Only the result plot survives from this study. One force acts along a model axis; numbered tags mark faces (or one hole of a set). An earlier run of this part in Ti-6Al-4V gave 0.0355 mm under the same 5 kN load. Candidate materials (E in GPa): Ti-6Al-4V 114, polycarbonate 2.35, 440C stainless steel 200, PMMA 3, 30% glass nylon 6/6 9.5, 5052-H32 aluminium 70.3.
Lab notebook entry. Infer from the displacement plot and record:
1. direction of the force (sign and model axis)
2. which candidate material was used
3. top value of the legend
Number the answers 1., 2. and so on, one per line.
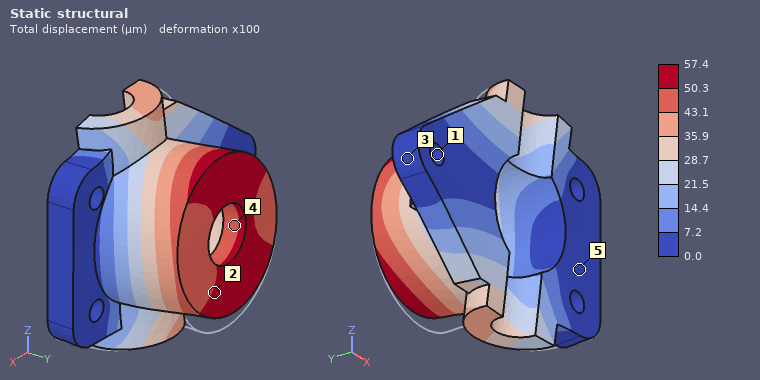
1. +Z
2. 5052-H32 aluminium
3. 57.4 µm
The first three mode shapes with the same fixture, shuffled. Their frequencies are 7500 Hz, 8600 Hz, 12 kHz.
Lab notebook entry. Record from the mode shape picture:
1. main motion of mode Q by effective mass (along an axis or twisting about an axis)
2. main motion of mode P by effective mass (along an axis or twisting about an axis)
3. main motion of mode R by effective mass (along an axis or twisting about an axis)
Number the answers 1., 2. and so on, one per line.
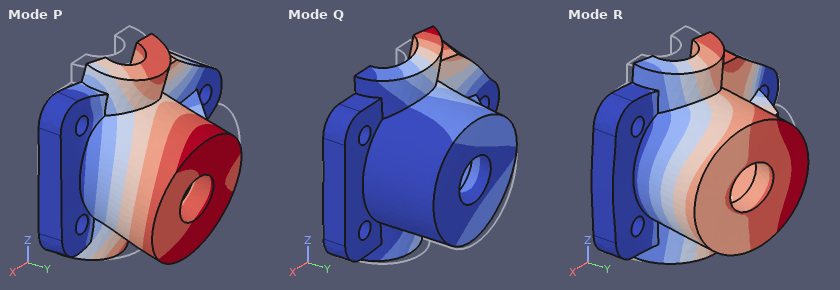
1. along Z
2. along Z
3. along Y
